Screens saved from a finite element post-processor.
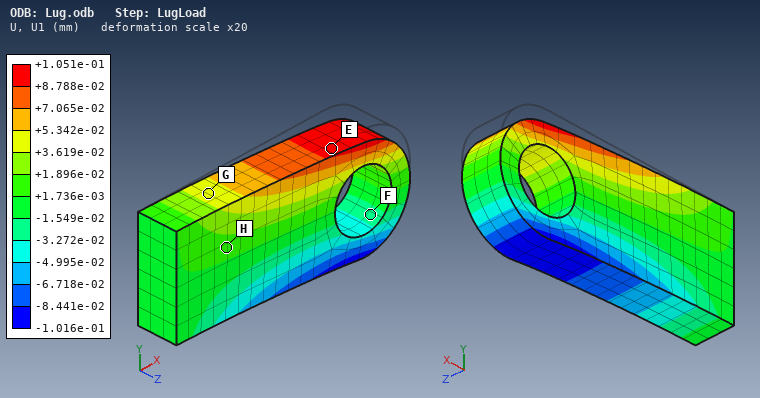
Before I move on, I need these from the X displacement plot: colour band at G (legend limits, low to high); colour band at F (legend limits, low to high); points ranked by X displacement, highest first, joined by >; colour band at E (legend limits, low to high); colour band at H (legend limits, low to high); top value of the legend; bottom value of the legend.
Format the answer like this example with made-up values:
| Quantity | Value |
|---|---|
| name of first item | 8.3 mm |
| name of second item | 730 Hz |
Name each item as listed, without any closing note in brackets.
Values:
| Quantity | Value |
|---|---|
| colour band at G | +3.619e-02 to +5.342e-02 mm |
| colour band at F | -3.272e-02 to -1.549e-02 mm |
| points ranked by X displacement, highest first, joined by > | E > G > H > F |
| colour band at E | +8.788e-02 to +1.051e-01 mm |
| colour band at H | +1.736e-03 to +1.896e-02 mm |
| top value of the legend | +1.051e-01 mm |
| bottom value of the legend | -1.016e-01 mm |
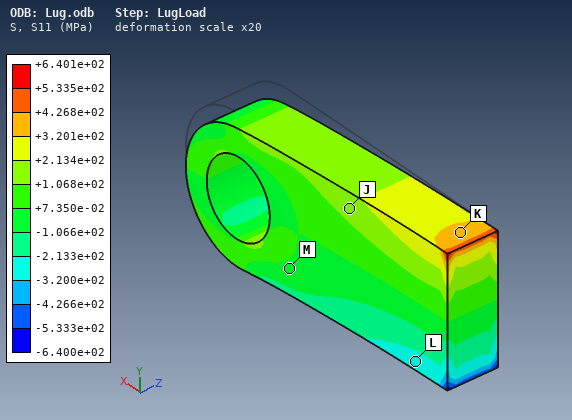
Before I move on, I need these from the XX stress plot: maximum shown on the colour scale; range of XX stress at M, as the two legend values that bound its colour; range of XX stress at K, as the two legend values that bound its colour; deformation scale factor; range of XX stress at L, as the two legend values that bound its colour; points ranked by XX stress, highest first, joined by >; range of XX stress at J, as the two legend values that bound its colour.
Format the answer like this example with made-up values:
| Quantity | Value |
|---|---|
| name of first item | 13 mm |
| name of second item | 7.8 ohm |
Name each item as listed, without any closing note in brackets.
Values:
| Quantity | Value |
|---|---|
| maximum shown on the colour scale | +6.401e+02 MPa |
| range of XX stress at M, as the two legend values that bound its colour | -1.066e+02 to +7.350e-02 MPa |
| range of XX stress at K, as the two legend values that bound its colour | +3.201e+02 to +4.268e+02 MPa |
| deformation scale factor | 20 |
| range of XX stress at L, as the two legend values that bound its colour | -3.200e+02 to -2.133e+02 MPa |
| points ranked by XX stress, highest first, joined by > | K > J > M > L |
| range of XX stress at J, as the two legend values that bound its colour | +1.068e+02 to +2.134e+02 MPa |
